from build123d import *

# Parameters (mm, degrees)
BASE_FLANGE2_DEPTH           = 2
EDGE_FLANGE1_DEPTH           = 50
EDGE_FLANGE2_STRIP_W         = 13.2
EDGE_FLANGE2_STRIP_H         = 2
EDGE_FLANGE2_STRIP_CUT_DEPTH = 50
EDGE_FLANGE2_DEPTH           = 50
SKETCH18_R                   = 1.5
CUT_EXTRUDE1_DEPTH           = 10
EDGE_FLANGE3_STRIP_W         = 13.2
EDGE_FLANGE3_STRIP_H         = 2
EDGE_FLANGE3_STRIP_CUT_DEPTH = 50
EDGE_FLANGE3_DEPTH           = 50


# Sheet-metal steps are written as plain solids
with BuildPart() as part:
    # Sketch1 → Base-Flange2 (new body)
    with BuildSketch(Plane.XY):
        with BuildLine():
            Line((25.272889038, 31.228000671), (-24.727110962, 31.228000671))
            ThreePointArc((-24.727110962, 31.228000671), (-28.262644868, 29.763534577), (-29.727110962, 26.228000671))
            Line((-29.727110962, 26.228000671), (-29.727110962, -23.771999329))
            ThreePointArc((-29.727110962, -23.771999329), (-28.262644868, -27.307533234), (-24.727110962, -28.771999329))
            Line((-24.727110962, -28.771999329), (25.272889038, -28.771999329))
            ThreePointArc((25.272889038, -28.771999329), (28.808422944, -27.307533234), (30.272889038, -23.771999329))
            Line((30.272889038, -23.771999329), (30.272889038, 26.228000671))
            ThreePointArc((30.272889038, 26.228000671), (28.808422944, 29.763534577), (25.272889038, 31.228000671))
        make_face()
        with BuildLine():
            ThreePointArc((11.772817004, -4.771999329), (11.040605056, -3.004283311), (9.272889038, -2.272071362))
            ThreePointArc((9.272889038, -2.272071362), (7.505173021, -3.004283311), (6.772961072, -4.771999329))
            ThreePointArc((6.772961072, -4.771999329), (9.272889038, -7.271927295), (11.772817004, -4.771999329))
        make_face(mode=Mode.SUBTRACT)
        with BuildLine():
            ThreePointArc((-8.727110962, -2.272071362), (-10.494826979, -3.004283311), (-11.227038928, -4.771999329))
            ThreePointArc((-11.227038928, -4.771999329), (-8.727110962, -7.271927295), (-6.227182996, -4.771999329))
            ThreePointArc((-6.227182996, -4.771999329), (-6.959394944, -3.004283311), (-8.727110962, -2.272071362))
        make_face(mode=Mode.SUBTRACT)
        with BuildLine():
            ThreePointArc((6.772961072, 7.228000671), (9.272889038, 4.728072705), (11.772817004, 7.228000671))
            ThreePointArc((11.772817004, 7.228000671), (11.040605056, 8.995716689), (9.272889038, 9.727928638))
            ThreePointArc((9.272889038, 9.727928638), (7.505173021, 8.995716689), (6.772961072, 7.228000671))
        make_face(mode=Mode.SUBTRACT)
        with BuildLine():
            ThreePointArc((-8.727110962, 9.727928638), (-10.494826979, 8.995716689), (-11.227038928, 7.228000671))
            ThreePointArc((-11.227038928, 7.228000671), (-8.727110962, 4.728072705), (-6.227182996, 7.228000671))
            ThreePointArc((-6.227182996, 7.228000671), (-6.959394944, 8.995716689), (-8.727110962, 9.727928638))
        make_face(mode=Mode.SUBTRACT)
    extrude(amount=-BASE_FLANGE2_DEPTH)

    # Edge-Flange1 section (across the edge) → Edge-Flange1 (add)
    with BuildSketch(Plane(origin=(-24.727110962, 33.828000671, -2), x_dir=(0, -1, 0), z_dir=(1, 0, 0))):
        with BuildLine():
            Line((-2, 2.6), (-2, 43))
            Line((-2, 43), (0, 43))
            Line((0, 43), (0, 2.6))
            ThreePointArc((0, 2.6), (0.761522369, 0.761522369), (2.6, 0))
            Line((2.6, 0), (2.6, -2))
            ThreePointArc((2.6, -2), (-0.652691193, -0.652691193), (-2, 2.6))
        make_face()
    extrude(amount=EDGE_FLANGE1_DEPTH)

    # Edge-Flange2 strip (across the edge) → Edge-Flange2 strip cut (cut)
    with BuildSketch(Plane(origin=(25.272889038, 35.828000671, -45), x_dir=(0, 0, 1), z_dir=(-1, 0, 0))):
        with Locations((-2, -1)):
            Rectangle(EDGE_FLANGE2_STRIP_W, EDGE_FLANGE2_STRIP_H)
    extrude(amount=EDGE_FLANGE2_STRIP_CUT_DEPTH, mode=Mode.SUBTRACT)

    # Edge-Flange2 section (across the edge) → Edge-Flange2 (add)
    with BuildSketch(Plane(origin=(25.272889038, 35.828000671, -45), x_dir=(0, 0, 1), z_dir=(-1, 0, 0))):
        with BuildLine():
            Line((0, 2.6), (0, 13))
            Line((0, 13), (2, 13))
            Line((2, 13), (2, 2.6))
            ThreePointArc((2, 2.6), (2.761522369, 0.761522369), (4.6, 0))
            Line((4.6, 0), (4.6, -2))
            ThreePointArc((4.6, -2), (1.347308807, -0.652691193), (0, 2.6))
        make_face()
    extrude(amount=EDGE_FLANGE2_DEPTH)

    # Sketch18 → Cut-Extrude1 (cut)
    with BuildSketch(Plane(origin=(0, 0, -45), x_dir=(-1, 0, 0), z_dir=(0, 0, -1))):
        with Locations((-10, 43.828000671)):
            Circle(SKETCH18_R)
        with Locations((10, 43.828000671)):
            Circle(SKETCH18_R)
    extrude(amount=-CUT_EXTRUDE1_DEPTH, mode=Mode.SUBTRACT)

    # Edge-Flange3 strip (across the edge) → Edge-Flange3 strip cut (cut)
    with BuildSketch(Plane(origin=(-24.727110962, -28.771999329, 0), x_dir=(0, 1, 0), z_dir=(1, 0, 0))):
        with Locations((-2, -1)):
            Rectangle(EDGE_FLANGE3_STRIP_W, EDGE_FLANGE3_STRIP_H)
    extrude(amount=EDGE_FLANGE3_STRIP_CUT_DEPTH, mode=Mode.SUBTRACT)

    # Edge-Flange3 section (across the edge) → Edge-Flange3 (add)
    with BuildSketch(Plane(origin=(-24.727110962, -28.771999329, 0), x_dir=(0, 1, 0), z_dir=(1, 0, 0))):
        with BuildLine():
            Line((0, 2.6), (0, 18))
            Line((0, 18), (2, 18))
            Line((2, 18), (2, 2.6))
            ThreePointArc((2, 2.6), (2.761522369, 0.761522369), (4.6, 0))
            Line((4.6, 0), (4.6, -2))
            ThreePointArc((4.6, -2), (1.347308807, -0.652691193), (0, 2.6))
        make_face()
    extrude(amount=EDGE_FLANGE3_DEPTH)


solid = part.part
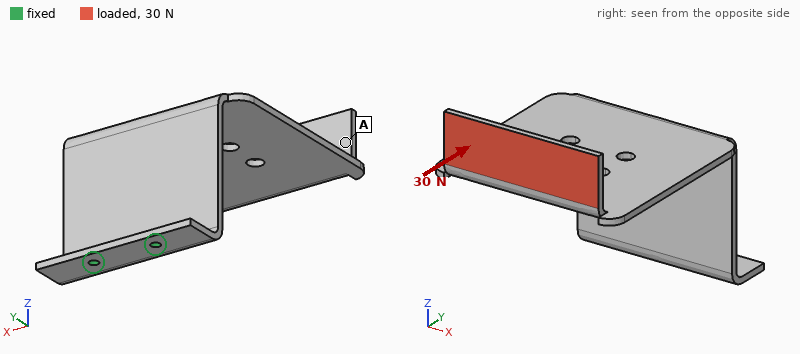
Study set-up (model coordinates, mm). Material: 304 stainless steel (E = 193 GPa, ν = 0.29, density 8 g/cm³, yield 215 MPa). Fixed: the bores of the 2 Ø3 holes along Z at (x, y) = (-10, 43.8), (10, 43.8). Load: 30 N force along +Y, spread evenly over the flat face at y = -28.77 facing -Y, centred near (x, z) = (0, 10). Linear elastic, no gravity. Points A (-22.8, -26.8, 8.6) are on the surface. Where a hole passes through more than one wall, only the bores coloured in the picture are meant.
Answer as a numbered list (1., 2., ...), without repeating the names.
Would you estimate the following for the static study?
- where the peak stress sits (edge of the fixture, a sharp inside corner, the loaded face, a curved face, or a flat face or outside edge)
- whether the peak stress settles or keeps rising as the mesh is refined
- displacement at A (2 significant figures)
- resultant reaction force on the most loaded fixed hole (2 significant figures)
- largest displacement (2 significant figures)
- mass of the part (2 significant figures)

1. edge of the fixture
2. keeps rising
3. 0.71 mm
4. 18 N
5. 0.79 mm
6. 110 g
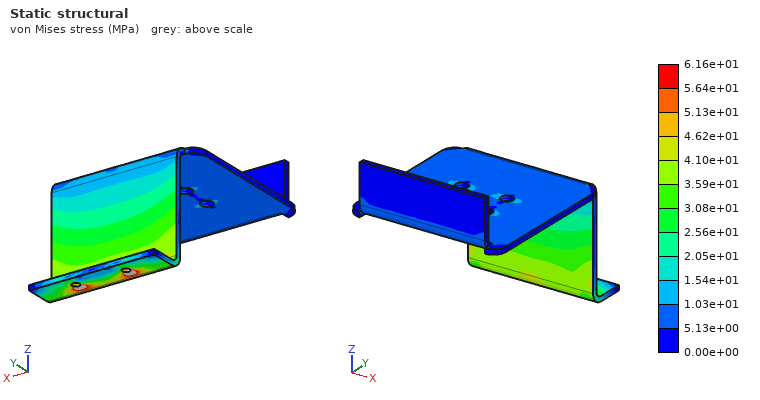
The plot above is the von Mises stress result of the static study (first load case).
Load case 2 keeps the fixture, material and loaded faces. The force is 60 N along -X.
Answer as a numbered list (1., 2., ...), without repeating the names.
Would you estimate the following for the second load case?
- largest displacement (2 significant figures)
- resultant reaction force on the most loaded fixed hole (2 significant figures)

1. 0.71 mm
2. 230 N
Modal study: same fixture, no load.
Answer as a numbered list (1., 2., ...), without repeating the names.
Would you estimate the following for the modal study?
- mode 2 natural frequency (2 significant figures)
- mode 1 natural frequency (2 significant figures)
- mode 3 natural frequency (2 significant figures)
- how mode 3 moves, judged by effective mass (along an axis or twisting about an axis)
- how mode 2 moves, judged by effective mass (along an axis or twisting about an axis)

1. 240 Hz
2. 120 Hz
3. 410 Hz
4. along Y
5. along X
